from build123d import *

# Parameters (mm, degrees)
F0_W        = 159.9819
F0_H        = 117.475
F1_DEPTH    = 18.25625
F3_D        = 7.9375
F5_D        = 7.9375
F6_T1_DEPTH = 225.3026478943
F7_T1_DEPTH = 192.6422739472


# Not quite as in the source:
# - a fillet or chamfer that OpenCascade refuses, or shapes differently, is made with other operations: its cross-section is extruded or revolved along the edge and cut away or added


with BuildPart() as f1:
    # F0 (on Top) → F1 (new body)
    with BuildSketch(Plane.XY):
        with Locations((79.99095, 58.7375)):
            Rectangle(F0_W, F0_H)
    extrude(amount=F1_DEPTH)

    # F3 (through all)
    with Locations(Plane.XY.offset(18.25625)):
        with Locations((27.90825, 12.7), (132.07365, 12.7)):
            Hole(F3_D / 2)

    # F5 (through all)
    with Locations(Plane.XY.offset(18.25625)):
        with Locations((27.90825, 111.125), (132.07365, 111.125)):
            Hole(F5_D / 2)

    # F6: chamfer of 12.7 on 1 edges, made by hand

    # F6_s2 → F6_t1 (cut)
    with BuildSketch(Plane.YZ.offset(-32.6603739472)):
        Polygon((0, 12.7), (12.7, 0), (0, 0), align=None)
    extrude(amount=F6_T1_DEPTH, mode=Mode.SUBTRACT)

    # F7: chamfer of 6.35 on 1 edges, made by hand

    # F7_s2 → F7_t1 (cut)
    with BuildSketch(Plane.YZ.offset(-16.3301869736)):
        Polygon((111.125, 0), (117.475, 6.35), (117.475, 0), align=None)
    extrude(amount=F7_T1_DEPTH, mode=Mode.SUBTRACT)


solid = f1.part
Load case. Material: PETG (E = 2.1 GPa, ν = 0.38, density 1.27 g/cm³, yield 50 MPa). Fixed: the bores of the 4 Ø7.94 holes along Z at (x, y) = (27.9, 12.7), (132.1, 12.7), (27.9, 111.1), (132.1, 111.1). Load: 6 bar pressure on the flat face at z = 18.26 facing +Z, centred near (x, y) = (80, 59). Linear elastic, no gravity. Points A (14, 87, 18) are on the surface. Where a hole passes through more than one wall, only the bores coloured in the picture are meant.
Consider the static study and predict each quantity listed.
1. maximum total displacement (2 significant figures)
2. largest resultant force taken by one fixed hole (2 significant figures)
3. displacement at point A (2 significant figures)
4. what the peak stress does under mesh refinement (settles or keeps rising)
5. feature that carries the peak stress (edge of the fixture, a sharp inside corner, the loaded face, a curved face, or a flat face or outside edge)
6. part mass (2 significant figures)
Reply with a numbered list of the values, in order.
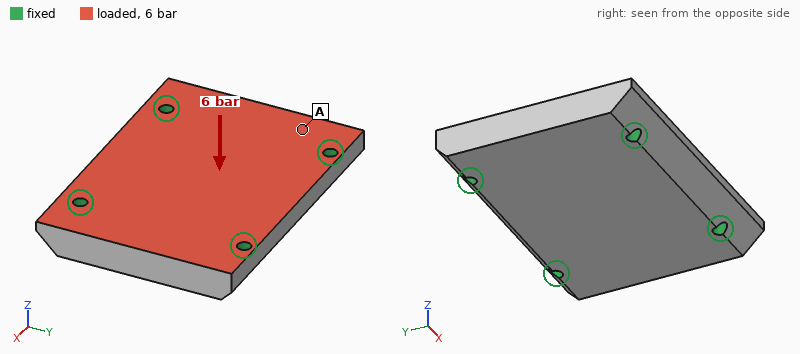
1. 0.53 mm
2. 3.0 kN
3. 0.22 mm
4. keeps rising
5. edge of the fixture
6. 410 g
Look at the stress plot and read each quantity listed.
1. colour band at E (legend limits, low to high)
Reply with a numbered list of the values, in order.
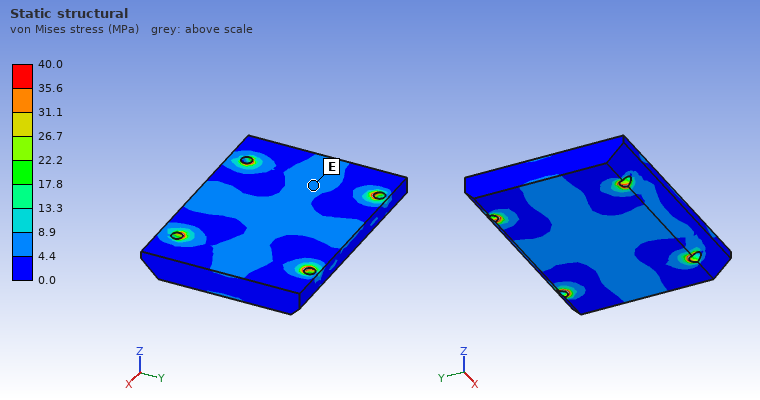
1. 4.4 to 8.9 MPa
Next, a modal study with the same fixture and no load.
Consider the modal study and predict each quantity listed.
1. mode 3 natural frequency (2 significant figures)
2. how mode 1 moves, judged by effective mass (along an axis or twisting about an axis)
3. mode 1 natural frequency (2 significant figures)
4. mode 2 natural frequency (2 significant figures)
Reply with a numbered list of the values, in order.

1. 1800 Hz
2. along Z
3. 1300 Hz
4. 1700 Hz
